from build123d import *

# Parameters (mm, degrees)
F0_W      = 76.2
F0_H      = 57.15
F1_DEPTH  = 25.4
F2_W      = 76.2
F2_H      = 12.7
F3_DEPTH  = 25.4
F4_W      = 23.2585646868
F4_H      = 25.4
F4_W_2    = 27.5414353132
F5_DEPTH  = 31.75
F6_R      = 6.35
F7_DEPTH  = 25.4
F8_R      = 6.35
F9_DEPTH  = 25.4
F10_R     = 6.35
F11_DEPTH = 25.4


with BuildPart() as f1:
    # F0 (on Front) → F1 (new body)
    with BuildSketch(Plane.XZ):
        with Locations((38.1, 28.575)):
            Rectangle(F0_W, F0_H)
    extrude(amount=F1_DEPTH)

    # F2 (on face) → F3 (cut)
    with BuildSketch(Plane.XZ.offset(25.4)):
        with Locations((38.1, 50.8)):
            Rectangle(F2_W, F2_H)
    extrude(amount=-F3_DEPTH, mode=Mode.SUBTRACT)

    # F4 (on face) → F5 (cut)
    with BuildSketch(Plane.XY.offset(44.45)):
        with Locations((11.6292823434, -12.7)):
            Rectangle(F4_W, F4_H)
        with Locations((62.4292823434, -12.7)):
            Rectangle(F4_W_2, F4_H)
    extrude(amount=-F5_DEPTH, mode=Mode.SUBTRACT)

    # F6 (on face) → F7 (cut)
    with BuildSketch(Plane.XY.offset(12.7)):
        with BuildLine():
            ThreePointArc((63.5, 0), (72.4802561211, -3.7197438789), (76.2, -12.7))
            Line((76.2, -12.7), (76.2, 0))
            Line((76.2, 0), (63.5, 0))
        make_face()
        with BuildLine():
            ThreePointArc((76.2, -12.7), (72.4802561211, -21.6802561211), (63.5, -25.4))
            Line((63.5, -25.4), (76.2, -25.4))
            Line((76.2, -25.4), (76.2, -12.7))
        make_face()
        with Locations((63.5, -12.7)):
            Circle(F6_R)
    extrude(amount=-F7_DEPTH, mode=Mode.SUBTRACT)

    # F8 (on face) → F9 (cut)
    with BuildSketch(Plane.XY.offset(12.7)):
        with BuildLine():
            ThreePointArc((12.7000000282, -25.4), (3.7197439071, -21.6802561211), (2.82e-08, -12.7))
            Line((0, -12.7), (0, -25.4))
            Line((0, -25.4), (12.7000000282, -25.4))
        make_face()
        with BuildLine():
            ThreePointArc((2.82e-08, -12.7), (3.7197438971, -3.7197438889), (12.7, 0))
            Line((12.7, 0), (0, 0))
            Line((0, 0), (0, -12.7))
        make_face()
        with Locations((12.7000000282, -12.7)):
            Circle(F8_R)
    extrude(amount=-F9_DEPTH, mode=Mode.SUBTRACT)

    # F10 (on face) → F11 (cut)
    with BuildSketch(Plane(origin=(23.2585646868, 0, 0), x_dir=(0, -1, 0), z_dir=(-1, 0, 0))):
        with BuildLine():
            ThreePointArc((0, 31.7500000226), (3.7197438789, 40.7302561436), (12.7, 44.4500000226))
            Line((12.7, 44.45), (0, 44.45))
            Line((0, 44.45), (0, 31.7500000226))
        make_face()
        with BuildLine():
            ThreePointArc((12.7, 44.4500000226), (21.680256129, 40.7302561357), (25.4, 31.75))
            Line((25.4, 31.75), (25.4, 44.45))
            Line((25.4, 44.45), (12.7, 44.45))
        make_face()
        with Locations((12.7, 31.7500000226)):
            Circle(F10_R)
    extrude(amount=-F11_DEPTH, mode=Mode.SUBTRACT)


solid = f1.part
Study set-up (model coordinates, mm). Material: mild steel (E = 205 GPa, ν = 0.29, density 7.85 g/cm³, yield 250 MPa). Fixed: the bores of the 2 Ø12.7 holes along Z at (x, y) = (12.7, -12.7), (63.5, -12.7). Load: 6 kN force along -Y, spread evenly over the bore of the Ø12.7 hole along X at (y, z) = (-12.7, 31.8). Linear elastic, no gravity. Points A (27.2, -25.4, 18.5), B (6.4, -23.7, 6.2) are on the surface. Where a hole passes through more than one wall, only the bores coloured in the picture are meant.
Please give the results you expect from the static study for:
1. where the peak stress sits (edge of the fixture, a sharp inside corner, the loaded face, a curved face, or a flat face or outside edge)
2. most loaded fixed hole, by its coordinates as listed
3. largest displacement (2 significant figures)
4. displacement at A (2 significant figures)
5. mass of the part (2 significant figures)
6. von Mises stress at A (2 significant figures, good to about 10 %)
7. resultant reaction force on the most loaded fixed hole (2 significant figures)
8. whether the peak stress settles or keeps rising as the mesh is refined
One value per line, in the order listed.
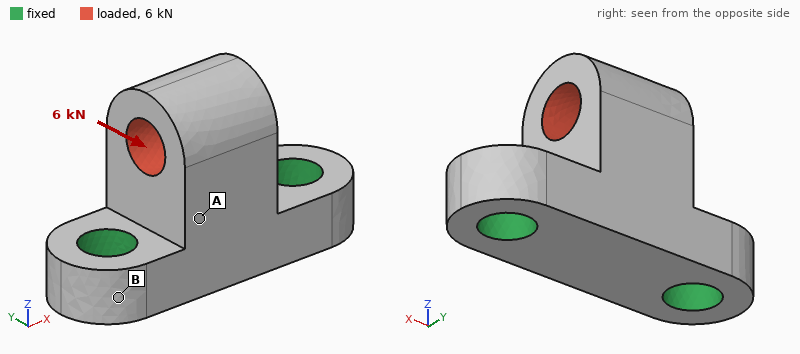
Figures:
edge of the fixture
(12.7, -12.7)
43 µm
17 µm
280 g
41 MPa
3.5 kN
keeps rising
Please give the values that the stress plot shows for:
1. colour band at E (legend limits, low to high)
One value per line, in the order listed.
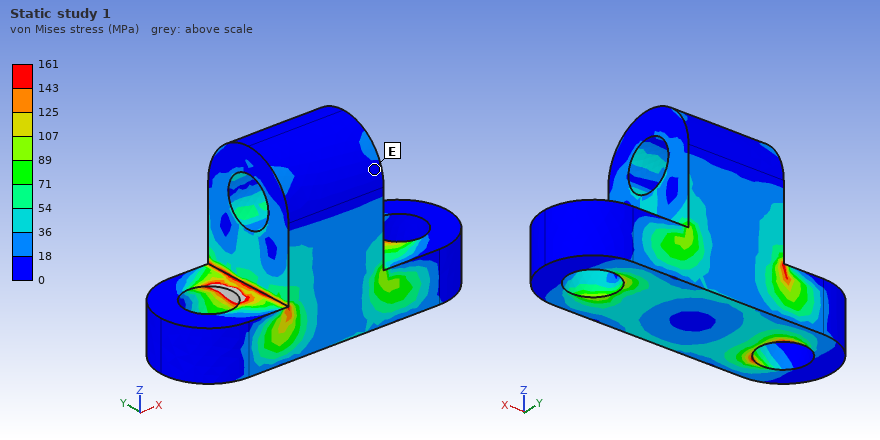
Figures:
0 to 18 MPa
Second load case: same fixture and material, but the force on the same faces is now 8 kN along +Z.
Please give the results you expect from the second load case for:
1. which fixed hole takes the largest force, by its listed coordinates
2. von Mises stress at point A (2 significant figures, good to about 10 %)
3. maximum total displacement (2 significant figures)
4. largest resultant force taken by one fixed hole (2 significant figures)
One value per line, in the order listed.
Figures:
(12.7, -12.7)
18 MPa
6.6 µm
4.5 kN
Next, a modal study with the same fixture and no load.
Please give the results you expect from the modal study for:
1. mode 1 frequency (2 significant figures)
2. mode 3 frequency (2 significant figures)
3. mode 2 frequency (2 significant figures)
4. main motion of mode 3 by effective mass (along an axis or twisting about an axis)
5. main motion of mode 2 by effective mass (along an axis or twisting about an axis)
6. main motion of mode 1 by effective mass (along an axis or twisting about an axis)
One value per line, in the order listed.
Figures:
7100 Hz
18 kHz
12 kHz
along Z
along X
along Y
